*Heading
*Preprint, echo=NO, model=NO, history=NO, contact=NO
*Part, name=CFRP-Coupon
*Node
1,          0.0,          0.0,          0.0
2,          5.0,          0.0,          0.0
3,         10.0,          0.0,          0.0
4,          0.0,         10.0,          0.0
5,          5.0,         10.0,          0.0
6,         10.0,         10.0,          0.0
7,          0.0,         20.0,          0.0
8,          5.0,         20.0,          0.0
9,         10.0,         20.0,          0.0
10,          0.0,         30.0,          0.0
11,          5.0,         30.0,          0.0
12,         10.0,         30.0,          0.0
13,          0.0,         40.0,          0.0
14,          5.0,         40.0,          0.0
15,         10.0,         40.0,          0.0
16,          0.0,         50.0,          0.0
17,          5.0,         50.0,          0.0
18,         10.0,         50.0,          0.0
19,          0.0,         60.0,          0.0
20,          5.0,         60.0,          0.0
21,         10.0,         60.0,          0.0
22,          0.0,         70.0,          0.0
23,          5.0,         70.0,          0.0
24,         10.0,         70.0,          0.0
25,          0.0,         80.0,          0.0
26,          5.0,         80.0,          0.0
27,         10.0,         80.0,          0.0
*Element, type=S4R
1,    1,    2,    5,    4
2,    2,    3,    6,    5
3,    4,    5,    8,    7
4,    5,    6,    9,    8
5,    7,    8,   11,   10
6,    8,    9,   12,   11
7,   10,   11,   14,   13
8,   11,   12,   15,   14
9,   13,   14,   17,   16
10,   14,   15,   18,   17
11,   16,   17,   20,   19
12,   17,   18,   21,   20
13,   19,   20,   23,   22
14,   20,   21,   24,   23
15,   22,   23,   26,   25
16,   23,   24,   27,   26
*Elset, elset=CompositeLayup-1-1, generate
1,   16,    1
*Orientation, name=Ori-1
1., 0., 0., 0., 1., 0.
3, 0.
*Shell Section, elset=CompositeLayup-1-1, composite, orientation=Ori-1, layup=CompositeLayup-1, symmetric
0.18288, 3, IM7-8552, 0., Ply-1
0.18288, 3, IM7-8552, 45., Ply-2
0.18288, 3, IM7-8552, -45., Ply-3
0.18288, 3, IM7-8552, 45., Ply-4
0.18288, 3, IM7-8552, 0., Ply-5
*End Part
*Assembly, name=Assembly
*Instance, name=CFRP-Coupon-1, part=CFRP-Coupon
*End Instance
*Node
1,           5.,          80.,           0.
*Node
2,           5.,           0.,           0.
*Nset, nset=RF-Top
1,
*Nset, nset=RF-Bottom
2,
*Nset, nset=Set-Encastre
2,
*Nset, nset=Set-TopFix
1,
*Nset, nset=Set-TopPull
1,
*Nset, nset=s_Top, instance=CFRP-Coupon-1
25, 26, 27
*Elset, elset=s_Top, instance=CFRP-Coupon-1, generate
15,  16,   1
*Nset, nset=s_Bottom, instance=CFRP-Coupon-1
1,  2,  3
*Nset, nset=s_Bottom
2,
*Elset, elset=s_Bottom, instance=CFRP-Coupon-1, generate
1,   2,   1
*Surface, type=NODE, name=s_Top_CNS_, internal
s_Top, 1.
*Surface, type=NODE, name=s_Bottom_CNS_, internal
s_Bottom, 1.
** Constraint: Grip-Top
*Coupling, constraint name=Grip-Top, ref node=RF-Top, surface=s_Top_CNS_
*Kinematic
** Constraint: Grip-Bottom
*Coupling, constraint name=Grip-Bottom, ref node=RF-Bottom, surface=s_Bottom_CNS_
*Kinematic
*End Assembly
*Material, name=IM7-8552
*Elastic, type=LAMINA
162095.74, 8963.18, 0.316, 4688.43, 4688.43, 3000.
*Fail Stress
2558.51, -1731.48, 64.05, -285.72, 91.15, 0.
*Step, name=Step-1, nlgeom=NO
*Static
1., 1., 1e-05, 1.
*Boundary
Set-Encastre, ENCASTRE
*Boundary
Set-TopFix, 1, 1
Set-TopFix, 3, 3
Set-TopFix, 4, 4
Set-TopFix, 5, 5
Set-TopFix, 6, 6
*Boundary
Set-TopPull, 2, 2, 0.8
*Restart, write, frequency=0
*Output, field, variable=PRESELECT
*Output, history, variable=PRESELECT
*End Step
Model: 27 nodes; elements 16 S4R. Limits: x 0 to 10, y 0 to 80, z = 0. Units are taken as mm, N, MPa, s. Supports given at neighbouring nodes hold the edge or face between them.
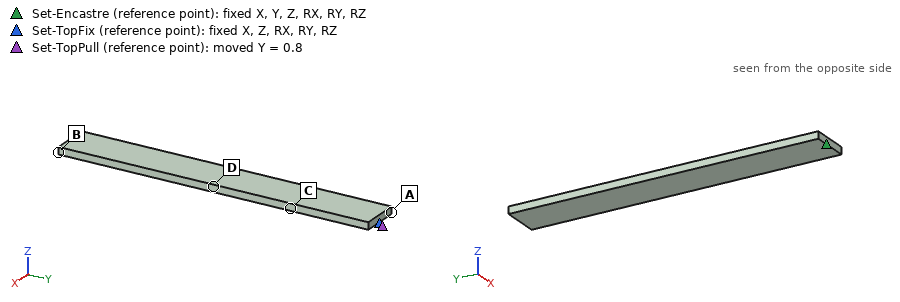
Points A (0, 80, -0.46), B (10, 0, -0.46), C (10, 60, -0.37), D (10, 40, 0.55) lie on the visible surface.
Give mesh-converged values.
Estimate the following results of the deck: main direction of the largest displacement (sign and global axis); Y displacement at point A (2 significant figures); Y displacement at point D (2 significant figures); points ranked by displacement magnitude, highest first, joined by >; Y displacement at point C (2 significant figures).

+Y
0.78 mm
0.38 mm
A > C > D > B
0.58 mm
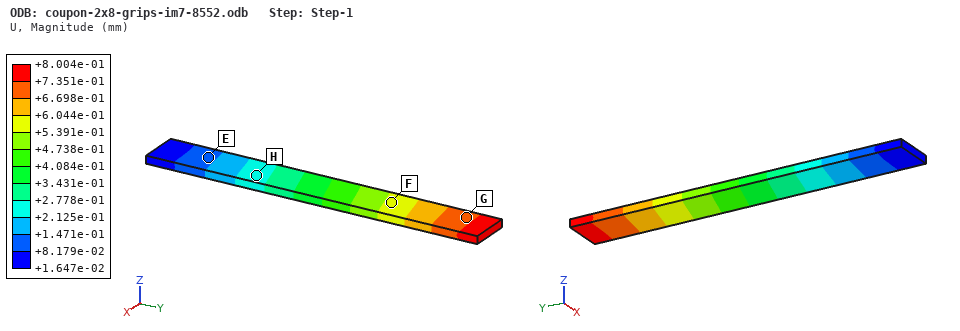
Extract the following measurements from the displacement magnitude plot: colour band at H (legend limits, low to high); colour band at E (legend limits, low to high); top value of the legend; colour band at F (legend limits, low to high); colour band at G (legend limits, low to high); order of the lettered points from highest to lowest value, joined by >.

+2.125e-01 to +2.778e-01 mm
+8.179e-02 to +1.471e-01 mm
+8.004e-01 mm
+5.391e-01 to +6.044e-01 mm
+6.698e-01 to +7.351e-01 mm
G > F > H > E
